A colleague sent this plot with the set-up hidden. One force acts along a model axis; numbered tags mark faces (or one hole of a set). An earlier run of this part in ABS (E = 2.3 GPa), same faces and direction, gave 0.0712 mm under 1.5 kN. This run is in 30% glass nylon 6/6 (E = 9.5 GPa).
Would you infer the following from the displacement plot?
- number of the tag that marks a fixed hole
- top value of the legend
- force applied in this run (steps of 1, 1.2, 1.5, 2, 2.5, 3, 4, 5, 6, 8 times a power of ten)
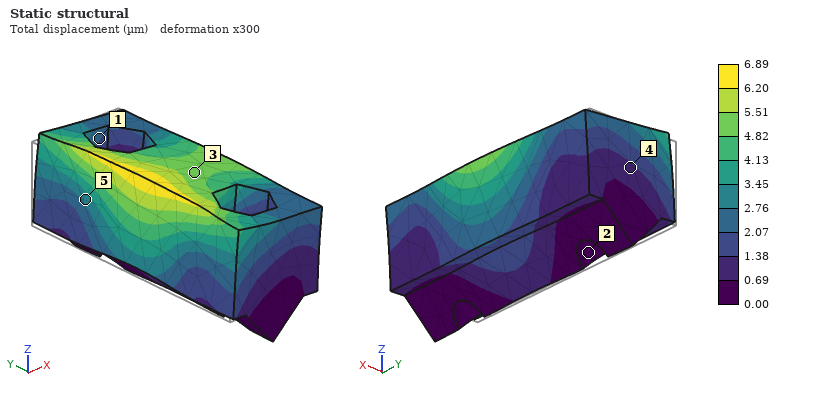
2
6.89 µm
600 N
